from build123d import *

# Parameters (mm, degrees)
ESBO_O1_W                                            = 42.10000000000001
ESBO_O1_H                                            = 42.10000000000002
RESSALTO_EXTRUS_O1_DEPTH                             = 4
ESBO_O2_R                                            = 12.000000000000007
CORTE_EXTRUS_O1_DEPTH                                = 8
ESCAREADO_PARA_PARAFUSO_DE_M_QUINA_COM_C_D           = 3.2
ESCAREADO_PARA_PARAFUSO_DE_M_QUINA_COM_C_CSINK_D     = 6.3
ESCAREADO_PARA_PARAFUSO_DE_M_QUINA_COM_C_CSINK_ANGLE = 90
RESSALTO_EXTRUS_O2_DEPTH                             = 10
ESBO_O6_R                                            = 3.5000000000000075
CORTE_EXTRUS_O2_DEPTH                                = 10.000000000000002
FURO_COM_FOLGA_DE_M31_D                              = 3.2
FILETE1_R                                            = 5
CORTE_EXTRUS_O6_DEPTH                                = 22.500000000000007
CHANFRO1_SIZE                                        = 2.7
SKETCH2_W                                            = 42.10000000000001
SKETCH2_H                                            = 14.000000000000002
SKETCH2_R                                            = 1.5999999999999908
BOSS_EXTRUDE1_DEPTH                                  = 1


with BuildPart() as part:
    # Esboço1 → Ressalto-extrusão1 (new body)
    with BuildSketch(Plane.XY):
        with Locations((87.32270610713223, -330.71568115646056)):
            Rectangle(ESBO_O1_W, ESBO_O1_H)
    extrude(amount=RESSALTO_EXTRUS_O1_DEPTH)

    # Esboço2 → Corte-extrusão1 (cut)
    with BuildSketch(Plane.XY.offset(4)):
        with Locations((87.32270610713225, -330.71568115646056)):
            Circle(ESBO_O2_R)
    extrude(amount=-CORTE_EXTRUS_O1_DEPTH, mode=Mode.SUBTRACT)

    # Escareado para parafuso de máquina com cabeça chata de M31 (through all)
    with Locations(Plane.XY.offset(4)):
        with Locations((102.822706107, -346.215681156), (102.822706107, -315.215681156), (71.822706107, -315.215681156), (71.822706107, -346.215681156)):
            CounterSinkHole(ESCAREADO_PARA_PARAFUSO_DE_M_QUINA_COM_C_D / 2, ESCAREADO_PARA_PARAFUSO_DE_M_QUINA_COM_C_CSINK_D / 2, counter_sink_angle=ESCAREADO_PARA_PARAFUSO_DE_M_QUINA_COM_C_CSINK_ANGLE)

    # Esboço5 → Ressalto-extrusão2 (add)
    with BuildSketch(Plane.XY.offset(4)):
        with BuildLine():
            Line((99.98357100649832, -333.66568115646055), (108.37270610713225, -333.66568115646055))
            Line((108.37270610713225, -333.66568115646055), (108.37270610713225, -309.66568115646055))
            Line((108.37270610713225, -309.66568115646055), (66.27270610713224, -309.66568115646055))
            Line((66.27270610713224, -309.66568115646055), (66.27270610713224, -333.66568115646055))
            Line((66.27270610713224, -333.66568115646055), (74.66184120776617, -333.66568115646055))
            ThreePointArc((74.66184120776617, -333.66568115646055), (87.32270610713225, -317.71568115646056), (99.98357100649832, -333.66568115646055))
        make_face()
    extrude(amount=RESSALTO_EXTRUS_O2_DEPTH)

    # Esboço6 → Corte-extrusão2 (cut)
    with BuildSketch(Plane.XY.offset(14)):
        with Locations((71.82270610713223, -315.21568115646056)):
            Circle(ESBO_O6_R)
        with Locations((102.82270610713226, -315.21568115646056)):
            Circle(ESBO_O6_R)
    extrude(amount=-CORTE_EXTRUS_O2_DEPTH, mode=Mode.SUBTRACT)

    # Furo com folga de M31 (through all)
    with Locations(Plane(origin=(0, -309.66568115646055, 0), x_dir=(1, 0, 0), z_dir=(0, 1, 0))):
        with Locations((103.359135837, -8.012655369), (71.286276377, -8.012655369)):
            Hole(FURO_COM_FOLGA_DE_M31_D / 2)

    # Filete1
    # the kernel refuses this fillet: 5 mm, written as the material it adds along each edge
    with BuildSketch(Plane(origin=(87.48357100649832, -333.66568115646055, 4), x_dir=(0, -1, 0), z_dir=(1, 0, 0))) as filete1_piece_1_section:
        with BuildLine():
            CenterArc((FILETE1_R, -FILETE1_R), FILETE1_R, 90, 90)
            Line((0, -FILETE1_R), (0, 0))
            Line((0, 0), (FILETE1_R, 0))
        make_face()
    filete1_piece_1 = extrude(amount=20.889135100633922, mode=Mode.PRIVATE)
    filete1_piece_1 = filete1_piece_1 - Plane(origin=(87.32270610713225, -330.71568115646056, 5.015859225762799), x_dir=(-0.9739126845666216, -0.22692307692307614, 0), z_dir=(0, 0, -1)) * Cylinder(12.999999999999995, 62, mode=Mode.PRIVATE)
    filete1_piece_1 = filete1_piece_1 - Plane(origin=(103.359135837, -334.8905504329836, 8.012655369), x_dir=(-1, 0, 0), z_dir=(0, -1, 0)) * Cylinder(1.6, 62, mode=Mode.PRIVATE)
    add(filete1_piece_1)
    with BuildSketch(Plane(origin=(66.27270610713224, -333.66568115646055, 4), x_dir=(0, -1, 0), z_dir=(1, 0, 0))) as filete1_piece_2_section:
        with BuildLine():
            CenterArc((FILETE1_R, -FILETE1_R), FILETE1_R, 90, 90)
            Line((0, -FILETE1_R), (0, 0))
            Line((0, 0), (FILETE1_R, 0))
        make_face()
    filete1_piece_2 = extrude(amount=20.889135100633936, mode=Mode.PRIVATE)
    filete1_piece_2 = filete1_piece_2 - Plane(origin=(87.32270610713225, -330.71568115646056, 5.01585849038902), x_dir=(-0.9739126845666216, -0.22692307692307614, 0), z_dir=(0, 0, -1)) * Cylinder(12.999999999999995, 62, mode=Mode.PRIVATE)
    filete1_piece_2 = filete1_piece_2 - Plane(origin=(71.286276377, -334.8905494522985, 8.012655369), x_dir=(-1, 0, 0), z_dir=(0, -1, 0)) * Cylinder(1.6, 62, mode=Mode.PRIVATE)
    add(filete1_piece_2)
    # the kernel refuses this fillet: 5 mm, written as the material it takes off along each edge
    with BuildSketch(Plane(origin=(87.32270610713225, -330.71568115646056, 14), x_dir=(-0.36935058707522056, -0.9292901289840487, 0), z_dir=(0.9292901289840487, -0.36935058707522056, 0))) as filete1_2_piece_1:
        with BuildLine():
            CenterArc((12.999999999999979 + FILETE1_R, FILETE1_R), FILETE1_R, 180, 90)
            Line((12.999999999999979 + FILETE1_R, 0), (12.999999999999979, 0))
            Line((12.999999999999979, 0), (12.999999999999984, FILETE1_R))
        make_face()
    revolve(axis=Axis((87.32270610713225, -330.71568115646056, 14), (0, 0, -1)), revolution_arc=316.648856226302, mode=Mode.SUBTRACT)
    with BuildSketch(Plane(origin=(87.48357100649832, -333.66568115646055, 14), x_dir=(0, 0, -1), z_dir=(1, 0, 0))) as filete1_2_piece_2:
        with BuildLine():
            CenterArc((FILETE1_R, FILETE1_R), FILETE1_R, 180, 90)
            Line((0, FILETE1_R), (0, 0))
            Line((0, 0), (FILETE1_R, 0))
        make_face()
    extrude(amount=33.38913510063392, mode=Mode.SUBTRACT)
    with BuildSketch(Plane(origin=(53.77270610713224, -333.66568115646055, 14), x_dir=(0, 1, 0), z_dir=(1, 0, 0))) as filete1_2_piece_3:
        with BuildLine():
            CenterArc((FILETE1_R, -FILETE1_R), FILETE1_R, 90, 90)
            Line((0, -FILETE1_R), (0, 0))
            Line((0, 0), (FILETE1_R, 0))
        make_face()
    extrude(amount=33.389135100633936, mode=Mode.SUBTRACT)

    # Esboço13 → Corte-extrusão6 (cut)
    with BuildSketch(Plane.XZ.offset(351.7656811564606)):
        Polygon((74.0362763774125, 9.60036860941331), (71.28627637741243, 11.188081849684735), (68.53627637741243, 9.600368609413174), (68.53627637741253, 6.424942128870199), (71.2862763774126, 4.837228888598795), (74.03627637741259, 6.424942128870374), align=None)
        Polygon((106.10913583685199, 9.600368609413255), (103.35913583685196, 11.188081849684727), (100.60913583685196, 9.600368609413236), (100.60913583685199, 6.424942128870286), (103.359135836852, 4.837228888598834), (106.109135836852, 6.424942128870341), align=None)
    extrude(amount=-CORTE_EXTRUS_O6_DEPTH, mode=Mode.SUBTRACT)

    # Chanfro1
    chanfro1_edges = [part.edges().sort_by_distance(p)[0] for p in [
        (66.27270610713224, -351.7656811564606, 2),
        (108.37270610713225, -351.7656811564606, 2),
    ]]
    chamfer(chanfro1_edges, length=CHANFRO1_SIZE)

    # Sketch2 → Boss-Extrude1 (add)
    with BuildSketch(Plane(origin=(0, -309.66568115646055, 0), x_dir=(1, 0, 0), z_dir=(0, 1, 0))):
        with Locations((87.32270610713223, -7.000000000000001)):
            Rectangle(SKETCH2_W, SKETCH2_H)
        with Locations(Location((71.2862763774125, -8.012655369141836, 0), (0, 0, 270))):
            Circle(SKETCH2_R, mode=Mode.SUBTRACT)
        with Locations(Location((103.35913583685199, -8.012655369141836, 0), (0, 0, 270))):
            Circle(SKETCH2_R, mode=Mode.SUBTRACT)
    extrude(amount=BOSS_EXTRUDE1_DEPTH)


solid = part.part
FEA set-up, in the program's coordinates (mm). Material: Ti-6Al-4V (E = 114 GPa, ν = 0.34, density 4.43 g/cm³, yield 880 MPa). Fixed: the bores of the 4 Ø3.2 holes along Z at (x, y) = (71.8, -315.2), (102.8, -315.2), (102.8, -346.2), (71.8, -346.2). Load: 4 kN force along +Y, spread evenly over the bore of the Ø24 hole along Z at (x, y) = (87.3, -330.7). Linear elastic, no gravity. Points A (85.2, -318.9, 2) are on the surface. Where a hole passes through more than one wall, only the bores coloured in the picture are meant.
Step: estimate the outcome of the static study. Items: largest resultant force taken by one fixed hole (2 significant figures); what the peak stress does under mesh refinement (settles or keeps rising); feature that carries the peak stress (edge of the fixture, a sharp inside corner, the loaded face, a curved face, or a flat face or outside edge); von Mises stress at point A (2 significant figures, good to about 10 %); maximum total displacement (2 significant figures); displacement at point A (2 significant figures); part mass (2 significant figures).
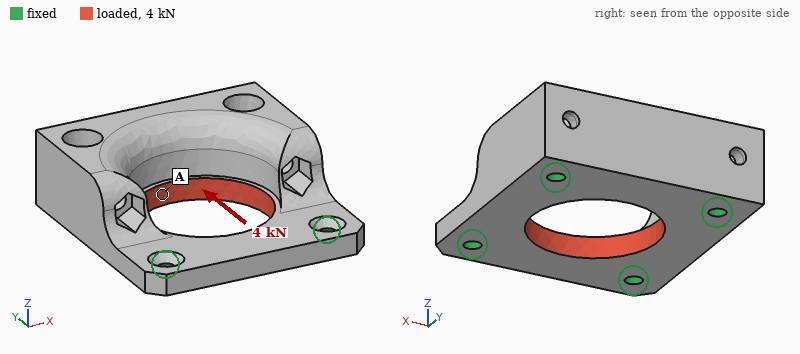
1.0 kN
keeps rising
edge of the fixture
13 MPa
7.2 µm
4.0 µm
48 g
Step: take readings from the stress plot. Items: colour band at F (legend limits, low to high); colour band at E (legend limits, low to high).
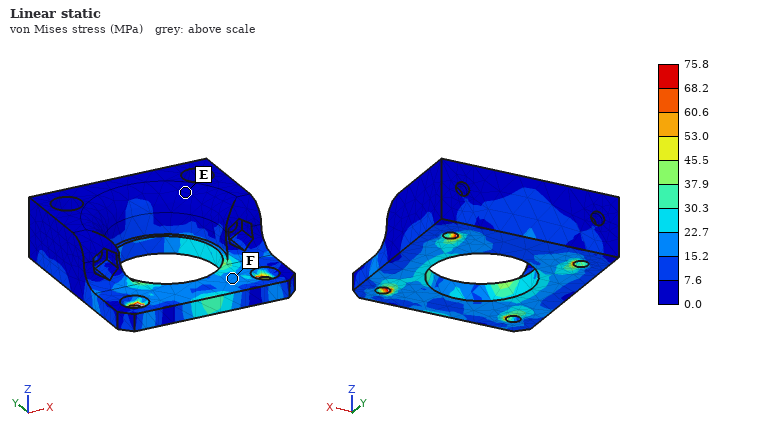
15.2 to 22.7 MPa
0.0 to 7.6 MPa
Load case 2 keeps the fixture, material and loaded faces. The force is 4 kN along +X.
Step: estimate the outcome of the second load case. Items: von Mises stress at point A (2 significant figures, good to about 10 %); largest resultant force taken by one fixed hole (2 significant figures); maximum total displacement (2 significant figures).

22 MPa
1.1 kN
5.3 µm
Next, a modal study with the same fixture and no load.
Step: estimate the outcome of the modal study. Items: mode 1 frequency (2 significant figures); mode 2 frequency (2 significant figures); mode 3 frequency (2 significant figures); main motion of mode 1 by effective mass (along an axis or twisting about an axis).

13 kHz
19 kHz
19 kHz
along Y
